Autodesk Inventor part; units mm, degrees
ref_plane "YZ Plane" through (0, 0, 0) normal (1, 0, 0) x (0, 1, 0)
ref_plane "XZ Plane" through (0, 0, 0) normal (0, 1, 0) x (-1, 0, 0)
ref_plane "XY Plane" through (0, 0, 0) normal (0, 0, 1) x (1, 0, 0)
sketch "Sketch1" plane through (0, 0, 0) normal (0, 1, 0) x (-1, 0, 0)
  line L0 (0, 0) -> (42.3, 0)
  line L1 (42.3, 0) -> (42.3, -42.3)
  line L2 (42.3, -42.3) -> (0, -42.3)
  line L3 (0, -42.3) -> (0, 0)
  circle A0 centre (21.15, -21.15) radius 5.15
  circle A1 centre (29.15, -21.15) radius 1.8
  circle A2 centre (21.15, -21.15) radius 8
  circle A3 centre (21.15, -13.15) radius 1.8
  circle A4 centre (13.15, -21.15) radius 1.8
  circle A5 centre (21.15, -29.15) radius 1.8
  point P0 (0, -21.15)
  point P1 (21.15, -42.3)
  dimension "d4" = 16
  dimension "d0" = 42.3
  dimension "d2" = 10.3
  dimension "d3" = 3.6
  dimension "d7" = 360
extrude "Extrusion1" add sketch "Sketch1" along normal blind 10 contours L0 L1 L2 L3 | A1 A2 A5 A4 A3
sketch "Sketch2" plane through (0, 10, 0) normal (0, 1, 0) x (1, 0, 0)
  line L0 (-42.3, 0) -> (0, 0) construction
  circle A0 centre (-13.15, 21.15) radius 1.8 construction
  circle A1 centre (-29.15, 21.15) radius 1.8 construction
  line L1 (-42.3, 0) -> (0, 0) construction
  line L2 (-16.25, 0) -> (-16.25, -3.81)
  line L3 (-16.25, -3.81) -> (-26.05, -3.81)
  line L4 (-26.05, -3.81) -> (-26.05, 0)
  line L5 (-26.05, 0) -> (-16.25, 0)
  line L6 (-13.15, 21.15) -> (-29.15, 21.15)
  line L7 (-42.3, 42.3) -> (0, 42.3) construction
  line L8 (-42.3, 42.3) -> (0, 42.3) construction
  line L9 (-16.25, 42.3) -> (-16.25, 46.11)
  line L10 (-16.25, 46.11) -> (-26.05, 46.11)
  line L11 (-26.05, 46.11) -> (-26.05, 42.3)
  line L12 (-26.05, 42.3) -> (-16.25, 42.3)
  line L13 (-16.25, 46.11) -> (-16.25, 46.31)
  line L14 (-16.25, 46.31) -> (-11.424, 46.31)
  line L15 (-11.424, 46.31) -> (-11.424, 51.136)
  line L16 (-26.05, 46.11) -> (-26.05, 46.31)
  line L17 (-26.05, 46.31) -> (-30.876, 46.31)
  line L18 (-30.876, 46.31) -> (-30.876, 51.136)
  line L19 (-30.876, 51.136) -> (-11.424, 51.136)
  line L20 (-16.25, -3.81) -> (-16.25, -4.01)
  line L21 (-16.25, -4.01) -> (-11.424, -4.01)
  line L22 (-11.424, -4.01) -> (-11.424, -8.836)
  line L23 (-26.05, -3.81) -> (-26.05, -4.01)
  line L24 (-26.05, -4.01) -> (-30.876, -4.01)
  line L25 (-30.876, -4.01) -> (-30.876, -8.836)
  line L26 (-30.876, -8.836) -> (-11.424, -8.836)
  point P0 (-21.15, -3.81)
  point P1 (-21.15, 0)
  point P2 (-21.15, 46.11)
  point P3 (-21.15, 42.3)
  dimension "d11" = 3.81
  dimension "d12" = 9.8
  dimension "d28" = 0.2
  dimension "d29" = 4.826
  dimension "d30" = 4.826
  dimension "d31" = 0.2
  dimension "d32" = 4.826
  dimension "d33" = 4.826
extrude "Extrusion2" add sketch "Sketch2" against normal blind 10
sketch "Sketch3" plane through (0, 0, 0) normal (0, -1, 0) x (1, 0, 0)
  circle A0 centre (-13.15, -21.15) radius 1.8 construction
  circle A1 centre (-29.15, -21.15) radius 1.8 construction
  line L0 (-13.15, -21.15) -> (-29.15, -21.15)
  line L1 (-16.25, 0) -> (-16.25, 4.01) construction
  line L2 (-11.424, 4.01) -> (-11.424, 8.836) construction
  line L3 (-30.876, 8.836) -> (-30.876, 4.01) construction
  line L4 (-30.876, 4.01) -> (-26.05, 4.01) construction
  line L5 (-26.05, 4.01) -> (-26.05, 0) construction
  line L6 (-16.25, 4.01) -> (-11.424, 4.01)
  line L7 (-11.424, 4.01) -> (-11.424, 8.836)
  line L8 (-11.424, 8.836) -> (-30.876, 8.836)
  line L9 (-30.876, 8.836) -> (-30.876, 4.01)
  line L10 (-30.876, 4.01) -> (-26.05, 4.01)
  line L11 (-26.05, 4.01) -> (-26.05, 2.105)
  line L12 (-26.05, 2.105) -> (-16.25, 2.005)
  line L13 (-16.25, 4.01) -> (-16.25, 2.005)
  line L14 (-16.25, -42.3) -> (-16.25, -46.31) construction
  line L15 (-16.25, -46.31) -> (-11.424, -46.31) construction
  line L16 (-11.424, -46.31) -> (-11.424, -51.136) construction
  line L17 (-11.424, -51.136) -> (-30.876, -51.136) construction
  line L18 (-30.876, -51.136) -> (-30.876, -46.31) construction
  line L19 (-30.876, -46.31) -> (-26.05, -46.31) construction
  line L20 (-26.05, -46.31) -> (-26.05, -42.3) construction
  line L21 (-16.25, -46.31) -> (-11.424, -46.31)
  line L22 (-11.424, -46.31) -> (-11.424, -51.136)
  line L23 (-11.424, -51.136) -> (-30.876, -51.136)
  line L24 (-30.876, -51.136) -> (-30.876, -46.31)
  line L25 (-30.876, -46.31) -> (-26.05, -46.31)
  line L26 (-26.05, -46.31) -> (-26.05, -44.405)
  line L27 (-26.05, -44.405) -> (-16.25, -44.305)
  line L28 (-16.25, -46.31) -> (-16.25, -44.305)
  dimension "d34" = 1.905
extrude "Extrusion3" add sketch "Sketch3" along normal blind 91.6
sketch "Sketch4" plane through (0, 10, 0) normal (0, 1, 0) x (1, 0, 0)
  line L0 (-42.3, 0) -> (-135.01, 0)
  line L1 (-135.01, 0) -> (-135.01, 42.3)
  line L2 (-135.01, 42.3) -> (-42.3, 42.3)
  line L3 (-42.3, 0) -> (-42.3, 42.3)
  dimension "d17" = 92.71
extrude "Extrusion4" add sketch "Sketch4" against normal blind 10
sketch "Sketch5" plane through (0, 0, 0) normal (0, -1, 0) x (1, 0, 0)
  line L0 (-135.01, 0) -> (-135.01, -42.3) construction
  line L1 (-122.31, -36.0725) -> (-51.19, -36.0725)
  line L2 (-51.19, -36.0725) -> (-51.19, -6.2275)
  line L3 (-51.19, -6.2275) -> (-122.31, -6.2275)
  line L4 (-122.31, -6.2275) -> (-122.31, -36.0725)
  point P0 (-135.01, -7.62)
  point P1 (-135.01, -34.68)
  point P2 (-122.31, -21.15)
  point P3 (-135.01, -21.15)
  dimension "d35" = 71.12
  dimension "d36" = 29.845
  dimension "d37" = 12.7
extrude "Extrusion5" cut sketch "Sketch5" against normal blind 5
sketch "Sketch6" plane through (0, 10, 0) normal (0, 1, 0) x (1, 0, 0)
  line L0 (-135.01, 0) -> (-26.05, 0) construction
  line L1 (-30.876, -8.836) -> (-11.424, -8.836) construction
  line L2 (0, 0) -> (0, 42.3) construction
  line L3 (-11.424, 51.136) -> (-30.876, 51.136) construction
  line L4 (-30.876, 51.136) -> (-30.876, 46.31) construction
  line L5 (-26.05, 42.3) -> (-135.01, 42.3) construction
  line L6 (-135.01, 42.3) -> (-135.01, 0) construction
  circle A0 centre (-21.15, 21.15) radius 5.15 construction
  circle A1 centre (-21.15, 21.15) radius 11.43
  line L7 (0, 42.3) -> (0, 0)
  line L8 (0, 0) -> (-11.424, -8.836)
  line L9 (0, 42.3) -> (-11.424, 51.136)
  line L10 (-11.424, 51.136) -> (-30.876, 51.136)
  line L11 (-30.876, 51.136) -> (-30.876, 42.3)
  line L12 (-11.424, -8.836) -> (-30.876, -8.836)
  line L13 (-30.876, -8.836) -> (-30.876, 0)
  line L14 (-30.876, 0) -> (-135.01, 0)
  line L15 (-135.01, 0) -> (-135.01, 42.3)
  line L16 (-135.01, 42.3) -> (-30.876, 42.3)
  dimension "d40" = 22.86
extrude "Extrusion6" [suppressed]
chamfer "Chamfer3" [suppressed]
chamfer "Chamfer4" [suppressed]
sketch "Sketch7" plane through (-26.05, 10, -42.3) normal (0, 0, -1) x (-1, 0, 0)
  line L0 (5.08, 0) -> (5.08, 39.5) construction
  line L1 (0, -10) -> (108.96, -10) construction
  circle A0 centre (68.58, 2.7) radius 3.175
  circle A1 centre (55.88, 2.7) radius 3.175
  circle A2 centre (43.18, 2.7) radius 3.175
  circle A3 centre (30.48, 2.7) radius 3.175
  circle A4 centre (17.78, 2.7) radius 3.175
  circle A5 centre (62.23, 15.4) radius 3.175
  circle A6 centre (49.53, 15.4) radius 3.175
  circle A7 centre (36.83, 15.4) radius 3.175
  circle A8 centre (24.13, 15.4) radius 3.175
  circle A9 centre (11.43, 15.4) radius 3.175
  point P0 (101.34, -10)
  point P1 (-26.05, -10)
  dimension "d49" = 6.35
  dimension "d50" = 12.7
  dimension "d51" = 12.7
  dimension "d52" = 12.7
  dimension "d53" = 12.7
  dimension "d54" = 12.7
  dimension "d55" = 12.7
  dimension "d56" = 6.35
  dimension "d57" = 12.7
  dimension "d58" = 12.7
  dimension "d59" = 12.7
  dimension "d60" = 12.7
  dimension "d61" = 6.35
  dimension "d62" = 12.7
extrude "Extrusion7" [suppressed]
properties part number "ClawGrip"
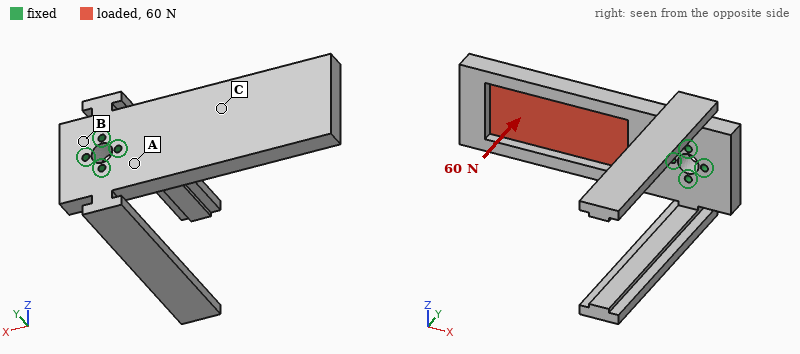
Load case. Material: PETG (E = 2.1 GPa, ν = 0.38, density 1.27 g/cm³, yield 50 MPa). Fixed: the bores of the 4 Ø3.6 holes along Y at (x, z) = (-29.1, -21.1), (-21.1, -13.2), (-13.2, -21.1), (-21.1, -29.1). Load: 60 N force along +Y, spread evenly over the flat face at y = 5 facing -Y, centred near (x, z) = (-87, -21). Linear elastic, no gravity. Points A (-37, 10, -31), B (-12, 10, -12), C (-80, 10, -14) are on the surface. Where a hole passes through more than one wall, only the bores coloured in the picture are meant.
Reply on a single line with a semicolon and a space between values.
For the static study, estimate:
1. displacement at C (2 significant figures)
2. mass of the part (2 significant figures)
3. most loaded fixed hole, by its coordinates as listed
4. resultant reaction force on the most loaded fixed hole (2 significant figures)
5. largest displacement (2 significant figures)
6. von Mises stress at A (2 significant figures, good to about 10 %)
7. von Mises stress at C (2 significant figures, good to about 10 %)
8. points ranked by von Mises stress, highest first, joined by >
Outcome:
0.67 mm; 87 g; (-29.1, -21.1); 160 N; 2.0 mm; 3.8 MPa; 1.5 MPa; A > C > B
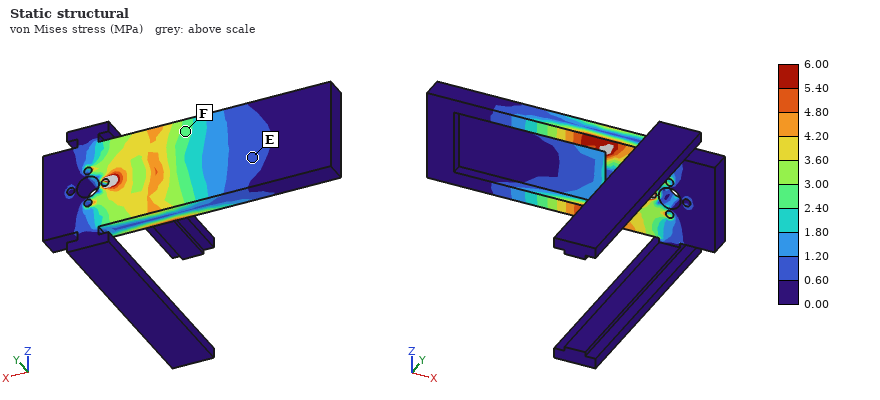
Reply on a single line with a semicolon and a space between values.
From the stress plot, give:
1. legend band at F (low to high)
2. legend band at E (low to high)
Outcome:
2.40 to 3.00 MPa; 0.60 to 1.20 MPa
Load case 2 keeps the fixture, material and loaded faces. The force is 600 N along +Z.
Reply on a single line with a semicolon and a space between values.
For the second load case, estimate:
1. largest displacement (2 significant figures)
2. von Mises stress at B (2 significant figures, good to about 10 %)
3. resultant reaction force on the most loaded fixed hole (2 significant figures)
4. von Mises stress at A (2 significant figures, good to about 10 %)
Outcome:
2.0 mm; 4.9 MPa; 1.3 kN; 6.5 MPa
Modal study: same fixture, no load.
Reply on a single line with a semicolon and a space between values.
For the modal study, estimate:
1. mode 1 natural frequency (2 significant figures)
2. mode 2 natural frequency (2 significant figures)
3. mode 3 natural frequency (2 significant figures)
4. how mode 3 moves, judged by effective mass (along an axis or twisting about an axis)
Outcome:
130 Hz; 130 Hz; 160 Hz; along Y
